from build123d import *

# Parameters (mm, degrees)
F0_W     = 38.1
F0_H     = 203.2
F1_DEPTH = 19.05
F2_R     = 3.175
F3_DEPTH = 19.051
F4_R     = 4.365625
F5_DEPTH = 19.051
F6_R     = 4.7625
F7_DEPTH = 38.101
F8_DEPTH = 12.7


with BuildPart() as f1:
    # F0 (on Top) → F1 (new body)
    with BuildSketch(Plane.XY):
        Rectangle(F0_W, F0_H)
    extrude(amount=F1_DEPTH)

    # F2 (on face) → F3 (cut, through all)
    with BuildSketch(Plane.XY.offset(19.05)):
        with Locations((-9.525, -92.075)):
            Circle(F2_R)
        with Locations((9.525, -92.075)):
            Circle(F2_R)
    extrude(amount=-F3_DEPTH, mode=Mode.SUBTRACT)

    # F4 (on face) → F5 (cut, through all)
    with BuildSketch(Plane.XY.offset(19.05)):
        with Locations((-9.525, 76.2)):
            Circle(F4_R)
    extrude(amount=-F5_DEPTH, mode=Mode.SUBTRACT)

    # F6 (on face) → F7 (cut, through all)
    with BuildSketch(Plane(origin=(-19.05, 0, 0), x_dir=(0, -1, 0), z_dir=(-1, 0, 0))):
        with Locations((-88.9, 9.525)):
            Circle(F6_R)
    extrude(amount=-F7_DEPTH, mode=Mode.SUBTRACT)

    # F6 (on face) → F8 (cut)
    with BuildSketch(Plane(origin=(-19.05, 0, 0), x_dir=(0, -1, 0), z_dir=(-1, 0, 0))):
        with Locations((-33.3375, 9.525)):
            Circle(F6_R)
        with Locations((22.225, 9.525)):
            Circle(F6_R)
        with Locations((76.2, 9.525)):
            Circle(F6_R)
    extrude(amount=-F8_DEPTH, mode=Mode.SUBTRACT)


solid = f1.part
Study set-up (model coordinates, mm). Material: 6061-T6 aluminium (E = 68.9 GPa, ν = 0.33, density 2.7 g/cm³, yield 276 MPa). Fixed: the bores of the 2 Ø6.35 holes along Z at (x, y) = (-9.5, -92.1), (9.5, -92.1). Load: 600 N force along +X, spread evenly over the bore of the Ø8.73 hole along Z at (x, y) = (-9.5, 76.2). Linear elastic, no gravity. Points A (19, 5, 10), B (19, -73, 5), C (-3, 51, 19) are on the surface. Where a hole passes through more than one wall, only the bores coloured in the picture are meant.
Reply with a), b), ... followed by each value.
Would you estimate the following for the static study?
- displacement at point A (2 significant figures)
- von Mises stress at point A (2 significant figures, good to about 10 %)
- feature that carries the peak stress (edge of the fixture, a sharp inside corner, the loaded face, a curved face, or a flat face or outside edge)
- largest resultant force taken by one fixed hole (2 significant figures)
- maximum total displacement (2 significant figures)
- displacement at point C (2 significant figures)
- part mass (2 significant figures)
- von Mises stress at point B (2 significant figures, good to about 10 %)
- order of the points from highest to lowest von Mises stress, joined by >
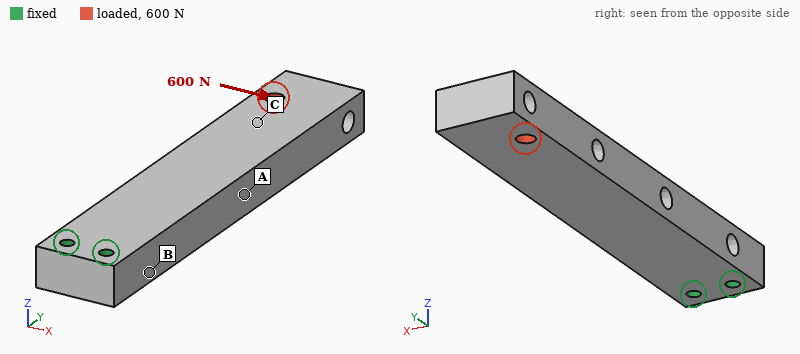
a) 0.084 mm
b) 9.5 MPa
c) a curved face
d) 4.4 kN
e) 0.24 mm
f) 0.15 mm
g) 380 g
h) 21 MPa
i) B > A > C
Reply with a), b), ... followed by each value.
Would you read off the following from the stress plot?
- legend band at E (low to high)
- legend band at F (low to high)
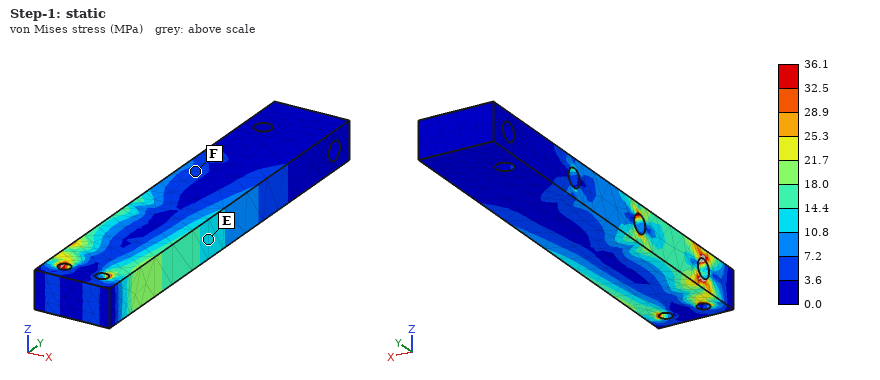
a) 10.8 to 14.4 MPa
b) 3.6 to 7.2 MPa
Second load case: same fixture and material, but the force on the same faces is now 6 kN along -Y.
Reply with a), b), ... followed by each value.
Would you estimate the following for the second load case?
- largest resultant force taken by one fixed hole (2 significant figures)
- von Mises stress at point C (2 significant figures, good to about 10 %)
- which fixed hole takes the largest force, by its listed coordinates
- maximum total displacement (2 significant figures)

a) 5.5 kN
b) 11 MPa
c) (-9.5, -92.1)
d) 0.23 mm
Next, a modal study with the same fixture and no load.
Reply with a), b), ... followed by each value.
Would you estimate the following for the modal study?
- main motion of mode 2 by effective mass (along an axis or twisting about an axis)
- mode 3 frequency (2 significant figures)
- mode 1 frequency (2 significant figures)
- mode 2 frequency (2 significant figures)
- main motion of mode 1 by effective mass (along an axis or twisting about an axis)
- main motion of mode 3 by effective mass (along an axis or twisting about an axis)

a) along X
b) 2500 Hz
c) 430 Hz
d) 780 Hz
e) along Z
f) along Z
